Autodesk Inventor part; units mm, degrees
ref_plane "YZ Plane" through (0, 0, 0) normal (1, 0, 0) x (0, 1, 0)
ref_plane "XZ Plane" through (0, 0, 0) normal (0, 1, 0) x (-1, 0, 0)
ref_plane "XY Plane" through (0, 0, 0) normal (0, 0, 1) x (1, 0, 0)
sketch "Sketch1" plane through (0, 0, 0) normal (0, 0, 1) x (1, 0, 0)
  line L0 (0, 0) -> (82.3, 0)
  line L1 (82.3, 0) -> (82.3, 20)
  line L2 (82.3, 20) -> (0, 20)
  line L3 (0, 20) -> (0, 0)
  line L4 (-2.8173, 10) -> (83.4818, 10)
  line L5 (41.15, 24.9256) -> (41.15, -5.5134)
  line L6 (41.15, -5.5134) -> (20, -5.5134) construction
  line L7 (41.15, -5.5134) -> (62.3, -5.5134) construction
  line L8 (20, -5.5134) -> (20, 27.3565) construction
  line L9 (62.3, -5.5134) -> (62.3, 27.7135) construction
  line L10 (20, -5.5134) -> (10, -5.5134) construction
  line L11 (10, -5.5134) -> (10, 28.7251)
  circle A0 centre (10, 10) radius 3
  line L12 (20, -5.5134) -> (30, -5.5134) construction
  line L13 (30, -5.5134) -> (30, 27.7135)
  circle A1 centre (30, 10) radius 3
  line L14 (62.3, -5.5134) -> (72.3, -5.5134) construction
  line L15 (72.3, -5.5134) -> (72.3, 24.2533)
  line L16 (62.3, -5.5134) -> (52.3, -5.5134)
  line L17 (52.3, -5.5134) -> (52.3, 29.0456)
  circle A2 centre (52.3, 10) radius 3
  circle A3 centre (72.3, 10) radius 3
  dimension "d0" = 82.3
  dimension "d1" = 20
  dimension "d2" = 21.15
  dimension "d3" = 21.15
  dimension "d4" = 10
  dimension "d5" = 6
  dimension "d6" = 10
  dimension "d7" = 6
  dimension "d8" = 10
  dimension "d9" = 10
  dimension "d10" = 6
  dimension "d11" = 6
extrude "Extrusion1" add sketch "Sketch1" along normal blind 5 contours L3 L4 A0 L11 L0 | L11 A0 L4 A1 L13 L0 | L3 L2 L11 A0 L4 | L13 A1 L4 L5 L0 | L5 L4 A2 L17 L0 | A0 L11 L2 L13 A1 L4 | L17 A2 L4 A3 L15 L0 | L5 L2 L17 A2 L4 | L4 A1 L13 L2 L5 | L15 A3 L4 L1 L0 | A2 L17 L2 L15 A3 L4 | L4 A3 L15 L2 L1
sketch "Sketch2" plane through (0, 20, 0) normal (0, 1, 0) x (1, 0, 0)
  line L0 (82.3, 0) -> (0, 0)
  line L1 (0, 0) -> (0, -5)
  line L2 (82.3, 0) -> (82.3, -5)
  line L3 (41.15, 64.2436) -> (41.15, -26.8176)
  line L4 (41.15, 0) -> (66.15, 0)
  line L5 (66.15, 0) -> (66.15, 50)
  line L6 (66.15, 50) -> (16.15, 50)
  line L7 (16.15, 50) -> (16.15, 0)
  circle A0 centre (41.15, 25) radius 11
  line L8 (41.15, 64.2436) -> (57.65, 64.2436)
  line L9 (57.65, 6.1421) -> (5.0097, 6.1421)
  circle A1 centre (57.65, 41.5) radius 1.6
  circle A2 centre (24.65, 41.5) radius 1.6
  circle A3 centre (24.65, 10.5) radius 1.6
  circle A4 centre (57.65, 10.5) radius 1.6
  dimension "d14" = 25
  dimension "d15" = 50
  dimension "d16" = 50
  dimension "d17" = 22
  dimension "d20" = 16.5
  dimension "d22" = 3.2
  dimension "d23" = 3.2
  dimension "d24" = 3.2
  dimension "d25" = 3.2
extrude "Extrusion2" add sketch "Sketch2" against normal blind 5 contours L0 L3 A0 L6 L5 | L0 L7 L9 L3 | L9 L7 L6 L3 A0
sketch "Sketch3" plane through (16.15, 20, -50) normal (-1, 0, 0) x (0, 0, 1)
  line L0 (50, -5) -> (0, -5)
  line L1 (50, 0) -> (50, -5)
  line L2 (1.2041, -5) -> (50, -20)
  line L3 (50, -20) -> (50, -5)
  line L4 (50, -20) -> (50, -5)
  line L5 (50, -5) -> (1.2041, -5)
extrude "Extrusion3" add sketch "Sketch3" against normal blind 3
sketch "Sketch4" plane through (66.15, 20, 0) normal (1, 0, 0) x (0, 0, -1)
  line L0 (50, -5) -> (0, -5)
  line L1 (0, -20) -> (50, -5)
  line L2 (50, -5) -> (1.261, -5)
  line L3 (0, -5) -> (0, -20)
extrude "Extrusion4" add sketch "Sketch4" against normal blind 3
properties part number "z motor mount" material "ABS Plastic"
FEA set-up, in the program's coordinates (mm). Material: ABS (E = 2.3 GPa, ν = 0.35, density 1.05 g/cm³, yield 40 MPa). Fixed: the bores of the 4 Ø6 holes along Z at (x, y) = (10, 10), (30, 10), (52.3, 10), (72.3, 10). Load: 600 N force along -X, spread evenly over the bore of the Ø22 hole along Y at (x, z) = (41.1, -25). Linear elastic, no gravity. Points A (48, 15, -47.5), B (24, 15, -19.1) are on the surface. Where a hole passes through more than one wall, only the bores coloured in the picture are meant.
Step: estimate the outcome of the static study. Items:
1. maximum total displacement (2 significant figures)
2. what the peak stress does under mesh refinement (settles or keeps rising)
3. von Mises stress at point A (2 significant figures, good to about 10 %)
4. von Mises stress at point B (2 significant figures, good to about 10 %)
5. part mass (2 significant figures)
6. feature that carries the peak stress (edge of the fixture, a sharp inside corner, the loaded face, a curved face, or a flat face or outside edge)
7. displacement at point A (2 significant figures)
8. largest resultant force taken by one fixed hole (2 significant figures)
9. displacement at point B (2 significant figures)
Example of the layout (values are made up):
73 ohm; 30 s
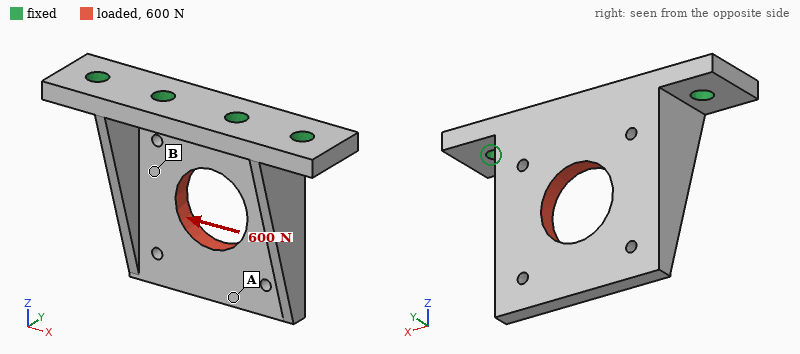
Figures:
0.63 mm; keeps rising; 2.3 MPa; 8.1 MPa; 21 g; edge of the fixture; 0.45 mm; 250 N; 0.24 mm
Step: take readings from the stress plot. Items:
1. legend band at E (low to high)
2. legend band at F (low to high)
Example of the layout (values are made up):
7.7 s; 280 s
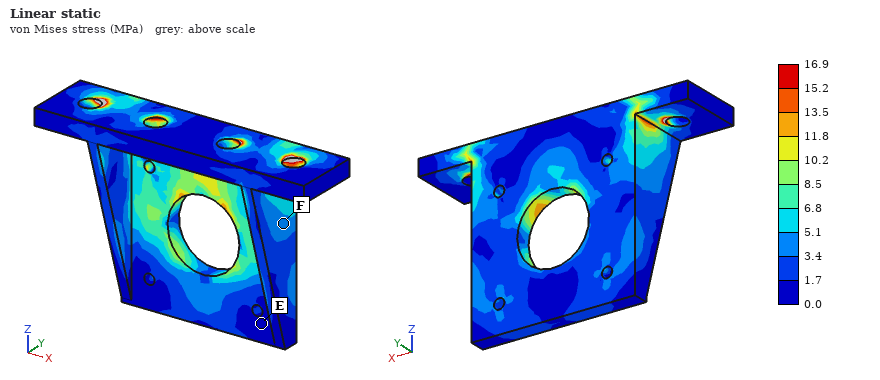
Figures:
0.0 to 1.7 MPa; 3.4 to 5.1 MPa
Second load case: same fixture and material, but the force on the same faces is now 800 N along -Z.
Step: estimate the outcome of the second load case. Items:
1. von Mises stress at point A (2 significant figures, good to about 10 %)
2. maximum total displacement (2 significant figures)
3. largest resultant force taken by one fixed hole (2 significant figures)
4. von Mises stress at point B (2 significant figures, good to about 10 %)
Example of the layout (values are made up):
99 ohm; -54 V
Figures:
2.8 MPa; 0.52 mm; 290 N; 3.5 MPa
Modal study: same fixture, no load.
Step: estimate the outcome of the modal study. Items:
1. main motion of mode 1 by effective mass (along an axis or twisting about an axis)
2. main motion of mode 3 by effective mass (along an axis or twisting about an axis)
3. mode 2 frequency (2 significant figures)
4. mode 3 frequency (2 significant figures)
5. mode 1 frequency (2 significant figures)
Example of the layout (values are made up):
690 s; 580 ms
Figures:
along Y; along X; 1200 Hz; 2400 Hz; 810 Hz
